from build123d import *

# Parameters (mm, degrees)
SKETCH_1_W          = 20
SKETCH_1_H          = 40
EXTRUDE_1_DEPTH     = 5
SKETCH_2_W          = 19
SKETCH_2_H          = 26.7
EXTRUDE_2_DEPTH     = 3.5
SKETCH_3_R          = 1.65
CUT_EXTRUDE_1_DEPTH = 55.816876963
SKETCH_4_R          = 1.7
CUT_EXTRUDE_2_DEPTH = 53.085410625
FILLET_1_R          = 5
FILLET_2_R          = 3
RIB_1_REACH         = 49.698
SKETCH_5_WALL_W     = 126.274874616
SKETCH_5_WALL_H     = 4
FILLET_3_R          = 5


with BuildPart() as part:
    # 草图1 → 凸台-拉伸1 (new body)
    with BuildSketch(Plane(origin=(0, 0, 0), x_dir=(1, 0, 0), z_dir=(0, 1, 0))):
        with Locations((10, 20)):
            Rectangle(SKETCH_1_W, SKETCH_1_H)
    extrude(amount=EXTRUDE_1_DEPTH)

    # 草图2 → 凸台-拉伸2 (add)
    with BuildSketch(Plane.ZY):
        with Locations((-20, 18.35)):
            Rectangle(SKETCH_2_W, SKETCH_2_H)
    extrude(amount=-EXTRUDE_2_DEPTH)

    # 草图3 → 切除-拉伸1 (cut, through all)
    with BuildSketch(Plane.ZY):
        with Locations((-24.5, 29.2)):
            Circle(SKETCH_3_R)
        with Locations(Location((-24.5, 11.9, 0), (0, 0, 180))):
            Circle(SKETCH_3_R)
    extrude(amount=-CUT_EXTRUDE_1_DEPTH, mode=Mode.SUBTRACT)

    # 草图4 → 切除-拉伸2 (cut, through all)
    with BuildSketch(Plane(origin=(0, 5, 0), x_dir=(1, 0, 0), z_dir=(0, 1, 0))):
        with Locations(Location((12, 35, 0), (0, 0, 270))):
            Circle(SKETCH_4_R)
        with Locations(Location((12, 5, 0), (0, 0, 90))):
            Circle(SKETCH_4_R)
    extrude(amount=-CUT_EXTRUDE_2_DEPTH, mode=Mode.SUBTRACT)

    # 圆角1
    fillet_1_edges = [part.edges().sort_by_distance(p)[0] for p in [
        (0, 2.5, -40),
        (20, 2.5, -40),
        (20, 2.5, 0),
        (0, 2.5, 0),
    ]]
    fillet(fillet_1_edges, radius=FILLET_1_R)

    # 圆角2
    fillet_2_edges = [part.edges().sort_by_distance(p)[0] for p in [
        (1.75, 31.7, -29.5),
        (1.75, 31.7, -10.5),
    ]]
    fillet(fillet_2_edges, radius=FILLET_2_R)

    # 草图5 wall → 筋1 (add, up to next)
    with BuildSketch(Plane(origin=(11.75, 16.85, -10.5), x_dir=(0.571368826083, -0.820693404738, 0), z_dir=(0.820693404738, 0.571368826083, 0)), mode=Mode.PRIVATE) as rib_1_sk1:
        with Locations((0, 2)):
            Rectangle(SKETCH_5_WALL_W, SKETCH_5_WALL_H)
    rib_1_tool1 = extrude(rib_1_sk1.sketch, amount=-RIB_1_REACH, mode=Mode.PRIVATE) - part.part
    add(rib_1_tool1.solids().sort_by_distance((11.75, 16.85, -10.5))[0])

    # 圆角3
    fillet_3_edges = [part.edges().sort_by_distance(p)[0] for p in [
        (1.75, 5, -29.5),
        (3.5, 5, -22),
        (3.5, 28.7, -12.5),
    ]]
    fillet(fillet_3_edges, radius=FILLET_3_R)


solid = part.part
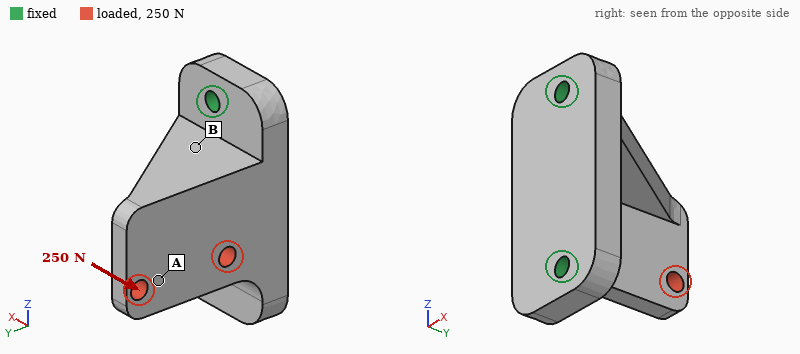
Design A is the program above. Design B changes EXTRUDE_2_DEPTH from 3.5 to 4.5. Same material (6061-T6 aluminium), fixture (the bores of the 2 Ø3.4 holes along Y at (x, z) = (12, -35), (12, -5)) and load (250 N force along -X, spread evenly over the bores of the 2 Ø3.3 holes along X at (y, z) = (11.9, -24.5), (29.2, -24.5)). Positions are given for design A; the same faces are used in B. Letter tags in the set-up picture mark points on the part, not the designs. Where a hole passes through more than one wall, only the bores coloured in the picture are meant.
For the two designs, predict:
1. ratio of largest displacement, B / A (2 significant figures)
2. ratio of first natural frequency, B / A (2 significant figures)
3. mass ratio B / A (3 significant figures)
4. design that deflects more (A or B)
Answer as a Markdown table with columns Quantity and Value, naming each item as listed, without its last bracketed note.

| Quantity | Value |
|---|---|
| ratio of largest displacement, B / A | 0.75 |
| ratio of first natural frequency, B / A | 0.96 |
| mass ratio B / A | 1.06 |
| design that deflects more | A |
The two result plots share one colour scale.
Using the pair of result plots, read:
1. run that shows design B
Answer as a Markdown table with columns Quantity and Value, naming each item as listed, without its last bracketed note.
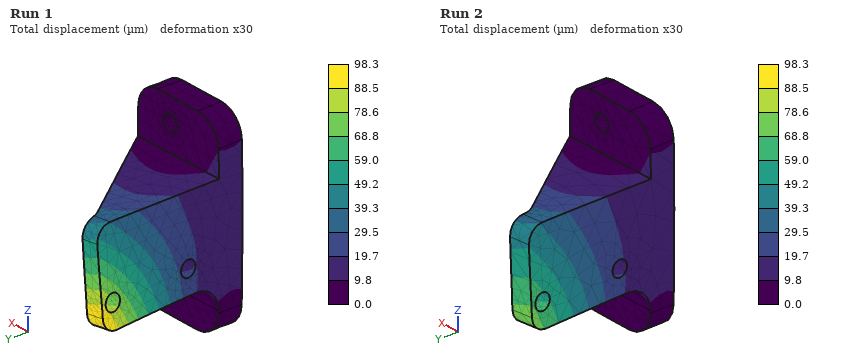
| Quantity | Value |
|---|---|
| run that shows design B | Run 2 |
